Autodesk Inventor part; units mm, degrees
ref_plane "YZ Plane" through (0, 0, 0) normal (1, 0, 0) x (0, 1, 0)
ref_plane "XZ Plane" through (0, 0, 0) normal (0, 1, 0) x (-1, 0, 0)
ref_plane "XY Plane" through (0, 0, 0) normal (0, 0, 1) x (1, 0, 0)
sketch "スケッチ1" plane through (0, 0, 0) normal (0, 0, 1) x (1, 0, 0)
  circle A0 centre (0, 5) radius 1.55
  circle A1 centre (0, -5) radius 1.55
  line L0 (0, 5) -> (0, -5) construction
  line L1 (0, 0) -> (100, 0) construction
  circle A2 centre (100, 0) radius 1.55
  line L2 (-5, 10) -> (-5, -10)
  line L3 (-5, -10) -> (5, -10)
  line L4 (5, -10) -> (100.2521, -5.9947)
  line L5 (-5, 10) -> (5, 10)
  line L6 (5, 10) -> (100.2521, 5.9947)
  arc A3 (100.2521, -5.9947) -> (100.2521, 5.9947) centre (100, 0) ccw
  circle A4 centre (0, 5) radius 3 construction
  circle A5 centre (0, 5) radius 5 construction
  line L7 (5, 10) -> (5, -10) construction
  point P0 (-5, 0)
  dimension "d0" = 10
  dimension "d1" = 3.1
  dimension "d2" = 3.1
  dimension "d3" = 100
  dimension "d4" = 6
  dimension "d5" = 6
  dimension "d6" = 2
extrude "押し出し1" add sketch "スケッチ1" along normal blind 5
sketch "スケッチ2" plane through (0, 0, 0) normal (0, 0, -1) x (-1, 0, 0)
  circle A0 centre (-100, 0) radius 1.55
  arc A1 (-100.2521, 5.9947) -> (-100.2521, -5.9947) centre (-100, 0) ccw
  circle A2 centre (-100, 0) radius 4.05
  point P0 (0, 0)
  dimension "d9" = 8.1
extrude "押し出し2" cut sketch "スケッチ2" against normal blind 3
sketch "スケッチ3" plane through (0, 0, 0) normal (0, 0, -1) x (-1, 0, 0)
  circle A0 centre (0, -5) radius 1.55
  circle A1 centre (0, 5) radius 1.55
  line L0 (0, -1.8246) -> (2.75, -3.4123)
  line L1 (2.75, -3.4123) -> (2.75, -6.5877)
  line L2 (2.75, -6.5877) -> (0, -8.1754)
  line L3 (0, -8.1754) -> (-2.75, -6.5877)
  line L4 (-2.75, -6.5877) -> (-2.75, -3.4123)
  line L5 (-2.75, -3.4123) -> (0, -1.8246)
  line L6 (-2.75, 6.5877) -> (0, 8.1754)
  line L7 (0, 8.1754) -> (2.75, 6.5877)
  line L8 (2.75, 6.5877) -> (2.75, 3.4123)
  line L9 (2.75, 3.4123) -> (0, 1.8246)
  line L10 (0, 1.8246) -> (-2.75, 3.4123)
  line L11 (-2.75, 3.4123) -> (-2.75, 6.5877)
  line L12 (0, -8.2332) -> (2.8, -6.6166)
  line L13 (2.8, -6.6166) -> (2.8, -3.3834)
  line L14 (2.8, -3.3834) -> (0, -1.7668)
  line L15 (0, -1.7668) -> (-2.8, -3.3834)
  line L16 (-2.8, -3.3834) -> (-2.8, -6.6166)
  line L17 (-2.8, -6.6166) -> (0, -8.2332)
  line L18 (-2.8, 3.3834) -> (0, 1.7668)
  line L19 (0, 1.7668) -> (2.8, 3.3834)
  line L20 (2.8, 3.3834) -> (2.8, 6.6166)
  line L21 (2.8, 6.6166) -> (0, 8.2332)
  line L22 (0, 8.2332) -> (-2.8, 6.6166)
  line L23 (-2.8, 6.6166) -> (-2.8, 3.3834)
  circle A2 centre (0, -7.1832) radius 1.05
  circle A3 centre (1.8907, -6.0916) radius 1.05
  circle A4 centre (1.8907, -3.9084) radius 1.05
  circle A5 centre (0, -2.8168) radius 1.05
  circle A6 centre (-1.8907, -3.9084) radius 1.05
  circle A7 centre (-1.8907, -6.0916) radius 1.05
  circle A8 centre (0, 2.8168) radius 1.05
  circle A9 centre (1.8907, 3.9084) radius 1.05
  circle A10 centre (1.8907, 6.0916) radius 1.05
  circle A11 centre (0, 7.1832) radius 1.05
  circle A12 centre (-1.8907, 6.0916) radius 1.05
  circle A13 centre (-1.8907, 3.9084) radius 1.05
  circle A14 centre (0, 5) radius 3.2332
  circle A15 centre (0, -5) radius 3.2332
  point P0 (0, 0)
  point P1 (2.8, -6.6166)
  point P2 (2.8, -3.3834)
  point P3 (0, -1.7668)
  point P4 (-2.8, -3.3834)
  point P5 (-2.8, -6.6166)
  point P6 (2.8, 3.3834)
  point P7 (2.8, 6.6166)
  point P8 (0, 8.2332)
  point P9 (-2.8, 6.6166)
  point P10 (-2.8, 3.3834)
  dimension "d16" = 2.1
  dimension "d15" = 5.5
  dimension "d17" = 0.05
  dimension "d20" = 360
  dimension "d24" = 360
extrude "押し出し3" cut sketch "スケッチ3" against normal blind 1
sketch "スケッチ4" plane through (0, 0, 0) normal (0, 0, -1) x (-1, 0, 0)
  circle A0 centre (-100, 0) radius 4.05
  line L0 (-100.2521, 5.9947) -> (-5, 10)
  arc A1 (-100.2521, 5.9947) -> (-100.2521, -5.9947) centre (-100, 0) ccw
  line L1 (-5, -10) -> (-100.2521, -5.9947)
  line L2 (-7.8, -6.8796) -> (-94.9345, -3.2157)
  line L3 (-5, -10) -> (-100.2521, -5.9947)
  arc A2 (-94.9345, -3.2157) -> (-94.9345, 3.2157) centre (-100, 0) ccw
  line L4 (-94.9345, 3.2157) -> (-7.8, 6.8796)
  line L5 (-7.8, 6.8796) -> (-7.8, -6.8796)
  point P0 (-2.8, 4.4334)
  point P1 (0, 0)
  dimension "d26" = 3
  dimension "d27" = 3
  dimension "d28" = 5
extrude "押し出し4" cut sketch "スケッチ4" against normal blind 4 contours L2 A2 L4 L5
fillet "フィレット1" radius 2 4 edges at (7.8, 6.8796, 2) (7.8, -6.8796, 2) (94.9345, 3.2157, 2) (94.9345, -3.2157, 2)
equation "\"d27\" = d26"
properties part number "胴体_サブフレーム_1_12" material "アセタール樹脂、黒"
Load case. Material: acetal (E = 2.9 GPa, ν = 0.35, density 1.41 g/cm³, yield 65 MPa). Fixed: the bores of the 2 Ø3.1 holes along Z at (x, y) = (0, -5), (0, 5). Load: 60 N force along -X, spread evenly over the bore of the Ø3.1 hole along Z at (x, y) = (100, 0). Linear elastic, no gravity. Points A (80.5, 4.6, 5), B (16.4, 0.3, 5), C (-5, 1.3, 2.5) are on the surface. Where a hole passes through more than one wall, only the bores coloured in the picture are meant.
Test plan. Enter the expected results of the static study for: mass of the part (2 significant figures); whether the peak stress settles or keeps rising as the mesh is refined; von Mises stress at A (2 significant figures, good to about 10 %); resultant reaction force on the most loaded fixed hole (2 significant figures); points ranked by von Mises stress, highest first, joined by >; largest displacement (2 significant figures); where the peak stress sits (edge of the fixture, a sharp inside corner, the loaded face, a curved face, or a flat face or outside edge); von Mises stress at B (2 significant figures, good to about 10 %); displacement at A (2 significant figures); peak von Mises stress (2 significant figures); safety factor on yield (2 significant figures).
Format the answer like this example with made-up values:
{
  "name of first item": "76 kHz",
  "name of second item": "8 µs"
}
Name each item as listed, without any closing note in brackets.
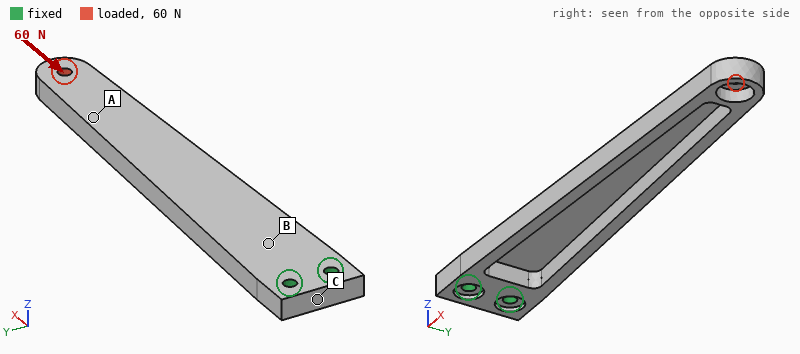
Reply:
{
  "mass of the part": "7.2 g",
  "whether the peak stress settles or keeps rising as the mesh is refined": "settles",
  "von Mises stress at A": "3.2 MPa",
  "resultant reaction force on the most loaded fixed hole": "30 N",
  "points ranked by von Mises stress, highest first, joined by >": "A > B > C",
  "largest displacement": "1.1 mm",
  "where the peak stress sits": "the loaded face",
  "von Mises stress at B": "2.6 MPa",
  "displacement at A": "0.61 mm",
  "peak von Mises stress": "6.5 MPa",
  "safety factor on yield": "10"
}
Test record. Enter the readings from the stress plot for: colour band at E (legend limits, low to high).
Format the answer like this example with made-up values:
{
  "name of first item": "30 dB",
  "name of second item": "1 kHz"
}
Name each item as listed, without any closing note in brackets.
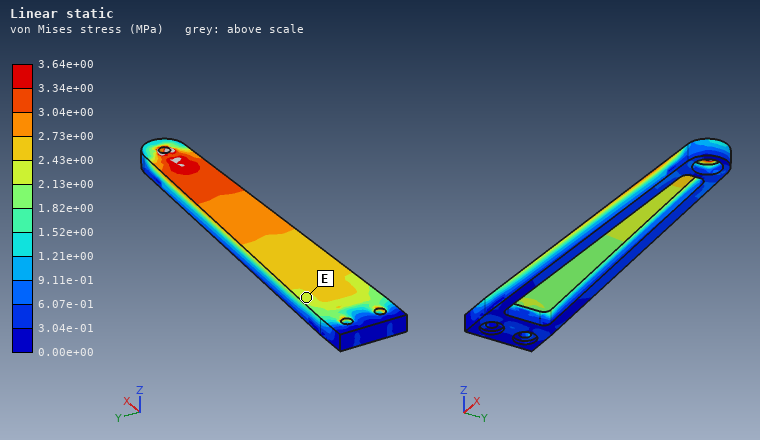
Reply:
{
  "colour band at E": "2.13e+00 to 2.43e+00 MPa"
}
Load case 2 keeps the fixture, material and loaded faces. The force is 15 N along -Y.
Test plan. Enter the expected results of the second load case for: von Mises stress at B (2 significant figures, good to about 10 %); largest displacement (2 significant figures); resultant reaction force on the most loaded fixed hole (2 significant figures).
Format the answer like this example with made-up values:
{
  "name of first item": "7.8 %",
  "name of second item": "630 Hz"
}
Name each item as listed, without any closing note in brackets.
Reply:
{
  "von Mises stress at B": "1.2 MPa",
  "largest displacement": "1.2 mm",
  "resultant reaction force on the most loaded fixed hole": "120 N"
}
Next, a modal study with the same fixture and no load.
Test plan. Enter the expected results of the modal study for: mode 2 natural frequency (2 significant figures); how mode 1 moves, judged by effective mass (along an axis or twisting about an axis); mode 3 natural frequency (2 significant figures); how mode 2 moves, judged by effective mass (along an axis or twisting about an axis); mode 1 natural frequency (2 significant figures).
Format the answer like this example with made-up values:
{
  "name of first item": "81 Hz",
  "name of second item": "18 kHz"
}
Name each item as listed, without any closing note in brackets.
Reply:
{
  "mode 2 natural frequency": "430 Hz",
  "how mode 1 moves, judged by effective mass": "along Z",
  "mode 3 natural frequency": "680 Hz",
  "how mode 2 moves, judged by effective mass": "along Y",
  "mode 1 natural frequency": "120 Hz"
}
